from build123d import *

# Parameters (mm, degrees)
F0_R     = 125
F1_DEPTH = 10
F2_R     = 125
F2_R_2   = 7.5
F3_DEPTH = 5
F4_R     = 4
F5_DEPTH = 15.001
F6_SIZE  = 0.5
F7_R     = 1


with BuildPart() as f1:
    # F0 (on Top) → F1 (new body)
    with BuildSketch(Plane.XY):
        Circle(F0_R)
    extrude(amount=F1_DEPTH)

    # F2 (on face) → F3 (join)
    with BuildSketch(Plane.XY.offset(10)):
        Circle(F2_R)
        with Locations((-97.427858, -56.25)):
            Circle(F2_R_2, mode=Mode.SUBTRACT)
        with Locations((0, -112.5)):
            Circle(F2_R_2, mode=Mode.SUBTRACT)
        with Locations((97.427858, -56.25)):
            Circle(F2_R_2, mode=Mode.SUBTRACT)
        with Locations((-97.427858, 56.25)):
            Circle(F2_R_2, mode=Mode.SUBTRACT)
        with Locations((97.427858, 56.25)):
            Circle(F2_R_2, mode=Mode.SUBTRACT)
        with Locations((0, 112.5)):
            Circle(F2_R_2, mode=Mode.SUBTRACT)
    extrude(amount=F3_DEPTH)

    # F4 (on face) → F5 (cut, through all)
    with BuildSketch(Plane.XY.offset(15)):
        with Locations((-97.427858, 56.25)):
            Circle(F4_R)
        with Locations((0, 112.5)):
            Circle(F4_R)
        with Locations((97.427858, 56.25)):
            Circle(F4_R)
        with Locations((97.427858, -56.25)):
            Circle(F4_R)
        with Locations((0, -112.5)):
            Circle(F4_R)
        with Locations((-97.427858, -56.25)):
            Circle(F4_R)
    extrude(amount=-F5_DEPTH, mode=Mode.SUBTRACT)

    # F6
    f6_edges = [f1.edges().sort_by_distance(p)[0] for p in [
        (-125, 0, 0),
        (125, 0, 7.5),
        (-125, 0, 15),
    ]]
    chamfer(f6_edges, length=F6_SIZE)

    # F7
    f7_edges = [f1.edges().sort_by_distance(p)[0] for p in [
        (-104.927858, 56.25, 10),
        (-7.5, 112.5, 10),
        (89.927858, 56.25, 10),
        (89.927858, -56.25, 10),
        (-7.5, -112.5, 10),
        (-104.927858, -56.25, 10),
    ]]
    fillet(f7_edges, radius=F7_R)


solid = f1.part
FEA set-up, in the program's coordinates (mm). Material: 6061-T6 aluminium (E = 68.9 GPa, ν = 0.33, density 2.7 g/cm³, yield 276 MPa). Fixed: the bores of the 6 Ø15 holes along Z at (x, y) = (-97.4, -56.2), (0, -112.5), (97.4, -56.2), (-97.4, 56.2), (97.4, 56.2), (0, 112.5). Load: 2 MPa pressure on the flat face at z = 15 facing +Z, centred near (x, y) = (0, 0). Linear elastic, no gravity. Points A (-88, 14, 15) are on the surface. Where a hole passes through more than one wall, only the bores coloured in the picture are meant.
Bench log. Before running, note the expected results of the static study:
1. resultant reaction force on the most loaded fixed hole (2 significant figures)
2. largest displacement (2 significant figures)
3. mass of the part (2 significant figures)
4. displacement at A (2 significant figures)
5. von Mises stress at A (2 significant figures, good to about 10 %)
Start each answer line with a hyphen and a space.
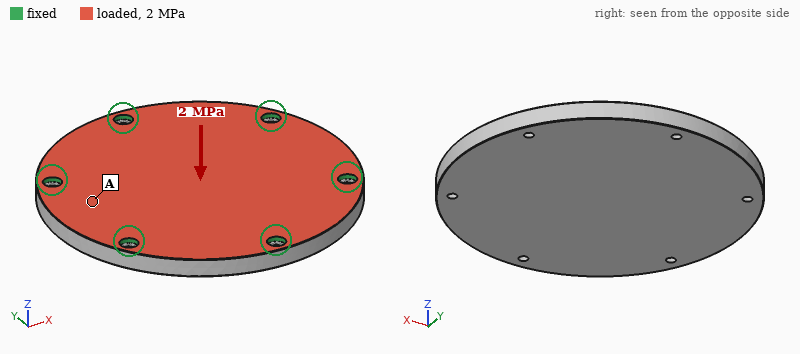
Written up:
- 21 kN
- 0.43 mm
- 2.0 kg
- 0.14 mm
- 38 MPa
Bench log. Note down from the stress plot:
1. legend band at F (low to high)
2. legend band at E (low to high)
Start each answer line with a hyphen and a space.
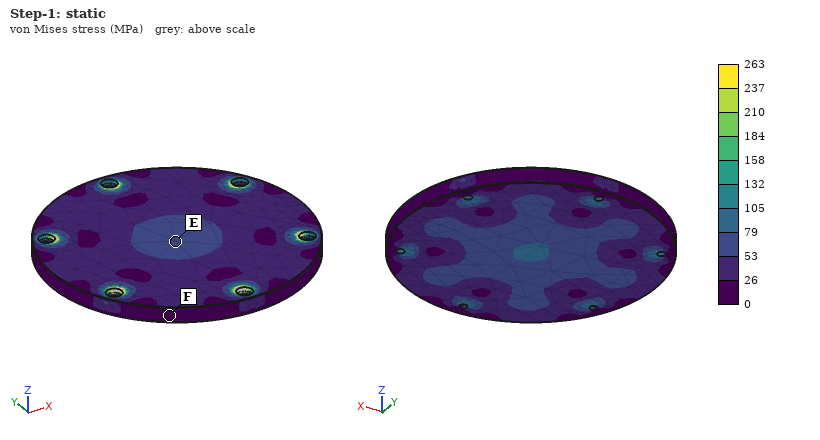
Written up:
- 0 to 26 MPa
- 53 to 79 MPa
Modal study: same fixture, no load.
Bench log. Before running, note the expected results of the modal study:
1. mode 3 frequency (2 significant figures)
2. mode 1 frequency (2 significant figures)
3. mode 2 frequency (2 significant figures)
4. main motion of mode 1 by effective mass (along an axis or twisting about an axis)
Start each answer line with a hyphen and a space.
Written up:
- 4200 Hz
- 2100 Hz
- 4200 Hz
- along Z
